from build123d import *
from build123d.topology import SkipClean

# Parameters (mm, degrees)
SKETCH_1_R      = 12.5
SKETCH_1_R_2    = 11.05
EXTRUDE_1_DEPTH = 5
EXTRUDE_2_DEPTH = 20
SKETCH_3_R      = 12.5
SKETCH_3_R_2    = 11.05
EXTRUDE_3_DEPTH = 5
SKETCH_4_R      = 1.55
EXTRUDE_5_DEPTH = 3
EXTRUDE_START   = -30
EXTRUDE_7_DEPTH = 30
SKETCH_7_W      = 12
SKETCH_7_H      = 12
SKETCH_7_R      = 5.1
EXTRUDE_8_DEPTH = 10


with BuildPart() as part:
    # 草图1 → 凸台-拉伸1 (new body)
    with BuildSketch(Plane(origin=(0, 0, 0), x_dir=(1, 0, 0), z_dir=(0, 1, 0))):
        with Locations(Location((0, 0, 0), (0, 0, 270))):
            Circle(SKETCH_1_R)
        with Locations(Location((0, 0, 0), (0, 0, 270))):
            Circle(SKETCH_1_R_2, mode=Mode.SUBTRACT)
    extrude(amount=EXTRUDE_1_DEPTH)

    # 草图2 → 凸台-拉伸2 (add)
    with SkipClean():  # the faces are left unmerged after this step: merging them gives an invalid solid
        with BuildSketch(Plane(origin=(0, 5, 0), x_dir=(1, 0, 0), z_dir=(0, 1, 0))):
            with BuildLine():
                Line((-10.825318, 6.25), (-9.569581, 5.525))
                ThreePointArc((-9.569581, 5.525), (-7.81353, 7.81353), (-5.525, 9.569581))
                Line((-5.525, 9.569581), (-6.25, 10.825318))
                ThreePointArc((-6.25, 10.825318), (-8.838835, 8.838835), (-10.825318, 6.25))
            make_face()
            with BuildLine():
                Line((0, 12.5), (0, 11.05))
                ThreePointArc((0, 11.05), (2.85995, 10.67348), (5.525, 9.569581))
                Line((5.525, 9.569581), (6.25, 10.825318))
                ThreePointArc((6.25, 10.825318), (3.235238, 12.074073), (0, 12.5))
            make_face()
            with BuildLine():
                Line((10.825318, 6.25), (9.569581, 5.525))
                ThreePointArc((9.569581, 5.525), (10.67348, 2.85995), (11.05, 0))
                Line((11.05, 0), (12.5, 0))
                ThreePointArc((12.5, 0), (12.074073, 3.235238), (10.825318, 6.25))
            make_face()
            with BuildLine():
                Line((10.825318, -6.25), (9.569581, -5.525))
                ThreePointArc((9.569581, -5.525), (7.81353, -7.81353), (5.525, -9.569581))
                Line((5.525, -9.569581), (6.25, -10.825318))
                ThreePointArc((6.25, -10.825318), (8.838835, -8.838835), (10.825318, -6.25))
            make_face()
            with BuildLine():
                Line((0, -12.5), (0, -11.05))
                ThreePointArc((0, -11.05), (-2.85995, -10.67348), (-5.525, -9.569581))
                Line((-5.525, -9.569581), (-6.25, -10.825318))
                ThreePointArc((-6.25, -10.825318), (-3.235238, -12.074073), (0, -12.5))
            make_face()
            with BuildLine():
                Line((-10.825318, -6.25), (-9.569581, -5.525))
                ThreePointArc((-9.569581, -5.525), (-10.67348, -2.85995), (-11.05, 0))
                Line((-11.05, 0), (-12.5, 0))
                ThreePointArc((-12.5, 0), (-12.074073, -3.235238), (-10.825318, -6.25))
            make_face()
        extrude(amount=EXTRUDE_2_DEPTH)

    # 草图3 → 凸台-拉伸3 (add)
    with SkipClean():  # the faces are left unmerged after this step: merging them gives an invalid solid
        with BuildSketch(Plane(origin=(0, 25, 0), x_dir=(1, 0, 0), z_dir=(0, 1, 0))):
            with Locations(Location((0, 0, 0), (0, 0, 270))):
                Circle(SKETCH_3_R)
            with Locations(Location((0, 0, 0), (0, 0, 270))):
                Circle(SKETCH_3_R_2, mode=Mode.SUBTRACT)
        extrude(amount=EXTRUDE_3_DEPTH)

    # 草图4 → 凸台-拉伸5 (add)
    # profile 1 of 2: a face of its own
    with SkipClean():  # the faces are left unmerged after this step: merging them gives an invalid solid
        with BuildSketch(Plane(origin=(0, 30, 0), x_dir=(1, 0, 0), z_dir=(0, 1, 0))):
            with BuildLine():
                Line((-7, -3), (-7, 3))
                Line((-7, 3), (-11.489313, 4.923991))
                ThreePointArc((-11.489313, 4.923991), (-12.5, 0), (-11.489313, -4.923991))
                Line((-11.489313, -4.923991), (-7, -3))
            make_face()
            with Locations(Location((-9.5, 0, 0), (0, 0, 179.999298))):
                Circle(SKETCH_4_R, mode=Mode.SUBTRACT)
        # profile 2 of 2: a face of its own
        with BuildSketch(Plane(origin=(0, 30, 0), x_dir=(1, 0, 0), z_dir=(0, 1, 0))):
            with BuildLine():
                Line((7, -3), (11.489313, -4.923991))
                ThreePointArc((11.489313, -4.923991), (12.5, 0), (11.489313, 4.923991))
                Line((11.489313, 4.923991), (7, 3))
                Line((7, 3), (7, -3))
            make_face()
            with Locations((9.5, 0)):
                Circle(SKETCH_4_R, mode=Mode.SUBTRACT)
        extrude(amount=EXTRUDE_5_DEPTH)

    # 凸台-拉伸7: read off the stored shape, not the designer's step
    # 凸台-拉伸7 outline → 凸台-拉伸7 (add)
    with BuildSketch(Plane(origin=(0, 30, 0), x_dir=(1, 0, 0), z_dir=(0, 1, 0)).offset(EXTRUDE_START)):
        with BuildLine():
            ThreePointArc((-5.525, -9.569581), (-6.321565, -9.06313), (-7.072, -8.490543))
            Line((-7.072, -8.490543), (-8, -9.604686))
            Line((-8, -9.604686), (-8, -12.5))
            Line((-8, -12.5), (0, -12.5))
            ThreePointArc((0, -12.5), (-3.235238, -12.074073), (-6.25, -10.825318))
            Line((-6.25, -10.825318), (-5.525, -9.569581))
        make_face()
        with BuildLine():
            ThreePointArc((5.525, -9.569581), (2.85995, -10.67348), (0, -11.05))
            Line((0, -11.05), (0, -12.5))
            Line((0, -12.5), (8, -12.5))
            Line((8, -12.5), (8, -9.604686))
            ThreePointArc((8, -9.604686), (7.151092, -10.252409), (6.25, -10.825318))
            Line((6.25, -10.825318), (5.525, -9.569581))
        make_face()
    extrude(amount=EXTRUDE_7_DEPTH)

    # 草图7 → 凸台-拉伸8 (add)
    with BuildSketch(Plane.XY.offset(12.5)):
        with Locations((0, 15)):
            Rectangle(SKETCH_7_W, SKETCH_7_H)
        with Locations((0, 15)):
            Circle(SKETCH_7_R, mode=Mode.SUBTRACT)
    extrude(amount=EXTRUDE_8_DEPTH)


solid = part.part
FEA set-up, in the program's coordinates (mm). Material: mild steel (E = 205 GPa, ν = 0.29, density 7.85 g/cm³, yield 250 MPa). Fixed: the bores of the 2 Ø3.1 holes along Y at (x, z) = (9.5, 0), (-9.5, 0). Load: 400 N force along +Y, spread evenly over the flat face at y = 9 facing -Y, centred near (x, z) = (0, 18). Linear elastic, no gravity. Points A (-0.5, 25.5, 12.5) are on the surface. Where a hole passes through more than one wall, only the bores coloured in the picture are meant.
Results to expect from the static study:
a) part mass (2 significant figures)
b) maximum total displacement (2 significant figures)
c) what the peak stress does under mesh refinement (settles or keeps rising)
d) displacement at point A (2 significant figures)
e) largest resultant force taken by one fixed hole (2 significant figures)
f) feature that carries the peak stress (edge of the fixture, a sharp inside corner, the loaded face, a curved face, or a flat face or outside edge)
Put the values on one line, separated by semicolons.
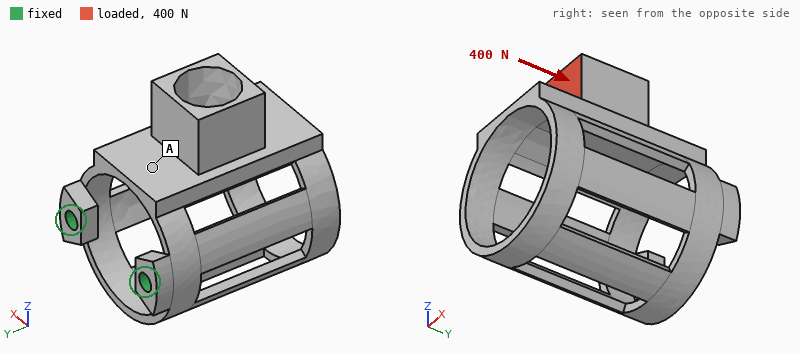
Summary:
29 g; 89 µm; keeps rising; 33 µm; 210 N; edge of the fixture
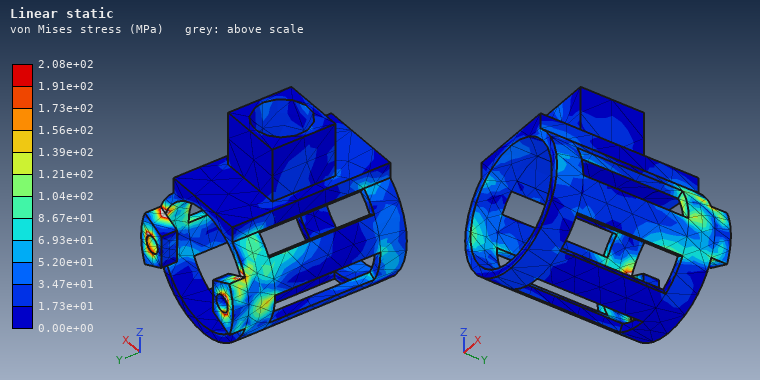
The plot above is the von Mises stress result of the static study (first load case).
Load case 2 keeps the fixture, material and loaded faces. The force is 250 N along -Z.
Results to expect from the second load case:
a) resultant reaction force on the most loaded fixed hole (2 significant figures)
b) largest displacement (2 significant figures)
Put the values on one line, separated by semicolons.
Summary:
130 N; 76 µm
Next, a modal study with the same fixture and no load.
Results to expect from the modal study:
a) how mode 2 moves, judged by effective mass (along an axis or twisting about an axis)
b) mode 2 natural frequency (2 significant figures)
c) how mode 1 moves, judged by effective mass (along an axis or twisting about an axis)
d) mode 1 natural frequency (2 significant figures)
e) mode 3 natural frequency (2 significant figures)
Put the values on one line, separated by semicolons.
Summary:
along X; 5000 Hz; along Z; 2400 Hz; 5900 Hz
